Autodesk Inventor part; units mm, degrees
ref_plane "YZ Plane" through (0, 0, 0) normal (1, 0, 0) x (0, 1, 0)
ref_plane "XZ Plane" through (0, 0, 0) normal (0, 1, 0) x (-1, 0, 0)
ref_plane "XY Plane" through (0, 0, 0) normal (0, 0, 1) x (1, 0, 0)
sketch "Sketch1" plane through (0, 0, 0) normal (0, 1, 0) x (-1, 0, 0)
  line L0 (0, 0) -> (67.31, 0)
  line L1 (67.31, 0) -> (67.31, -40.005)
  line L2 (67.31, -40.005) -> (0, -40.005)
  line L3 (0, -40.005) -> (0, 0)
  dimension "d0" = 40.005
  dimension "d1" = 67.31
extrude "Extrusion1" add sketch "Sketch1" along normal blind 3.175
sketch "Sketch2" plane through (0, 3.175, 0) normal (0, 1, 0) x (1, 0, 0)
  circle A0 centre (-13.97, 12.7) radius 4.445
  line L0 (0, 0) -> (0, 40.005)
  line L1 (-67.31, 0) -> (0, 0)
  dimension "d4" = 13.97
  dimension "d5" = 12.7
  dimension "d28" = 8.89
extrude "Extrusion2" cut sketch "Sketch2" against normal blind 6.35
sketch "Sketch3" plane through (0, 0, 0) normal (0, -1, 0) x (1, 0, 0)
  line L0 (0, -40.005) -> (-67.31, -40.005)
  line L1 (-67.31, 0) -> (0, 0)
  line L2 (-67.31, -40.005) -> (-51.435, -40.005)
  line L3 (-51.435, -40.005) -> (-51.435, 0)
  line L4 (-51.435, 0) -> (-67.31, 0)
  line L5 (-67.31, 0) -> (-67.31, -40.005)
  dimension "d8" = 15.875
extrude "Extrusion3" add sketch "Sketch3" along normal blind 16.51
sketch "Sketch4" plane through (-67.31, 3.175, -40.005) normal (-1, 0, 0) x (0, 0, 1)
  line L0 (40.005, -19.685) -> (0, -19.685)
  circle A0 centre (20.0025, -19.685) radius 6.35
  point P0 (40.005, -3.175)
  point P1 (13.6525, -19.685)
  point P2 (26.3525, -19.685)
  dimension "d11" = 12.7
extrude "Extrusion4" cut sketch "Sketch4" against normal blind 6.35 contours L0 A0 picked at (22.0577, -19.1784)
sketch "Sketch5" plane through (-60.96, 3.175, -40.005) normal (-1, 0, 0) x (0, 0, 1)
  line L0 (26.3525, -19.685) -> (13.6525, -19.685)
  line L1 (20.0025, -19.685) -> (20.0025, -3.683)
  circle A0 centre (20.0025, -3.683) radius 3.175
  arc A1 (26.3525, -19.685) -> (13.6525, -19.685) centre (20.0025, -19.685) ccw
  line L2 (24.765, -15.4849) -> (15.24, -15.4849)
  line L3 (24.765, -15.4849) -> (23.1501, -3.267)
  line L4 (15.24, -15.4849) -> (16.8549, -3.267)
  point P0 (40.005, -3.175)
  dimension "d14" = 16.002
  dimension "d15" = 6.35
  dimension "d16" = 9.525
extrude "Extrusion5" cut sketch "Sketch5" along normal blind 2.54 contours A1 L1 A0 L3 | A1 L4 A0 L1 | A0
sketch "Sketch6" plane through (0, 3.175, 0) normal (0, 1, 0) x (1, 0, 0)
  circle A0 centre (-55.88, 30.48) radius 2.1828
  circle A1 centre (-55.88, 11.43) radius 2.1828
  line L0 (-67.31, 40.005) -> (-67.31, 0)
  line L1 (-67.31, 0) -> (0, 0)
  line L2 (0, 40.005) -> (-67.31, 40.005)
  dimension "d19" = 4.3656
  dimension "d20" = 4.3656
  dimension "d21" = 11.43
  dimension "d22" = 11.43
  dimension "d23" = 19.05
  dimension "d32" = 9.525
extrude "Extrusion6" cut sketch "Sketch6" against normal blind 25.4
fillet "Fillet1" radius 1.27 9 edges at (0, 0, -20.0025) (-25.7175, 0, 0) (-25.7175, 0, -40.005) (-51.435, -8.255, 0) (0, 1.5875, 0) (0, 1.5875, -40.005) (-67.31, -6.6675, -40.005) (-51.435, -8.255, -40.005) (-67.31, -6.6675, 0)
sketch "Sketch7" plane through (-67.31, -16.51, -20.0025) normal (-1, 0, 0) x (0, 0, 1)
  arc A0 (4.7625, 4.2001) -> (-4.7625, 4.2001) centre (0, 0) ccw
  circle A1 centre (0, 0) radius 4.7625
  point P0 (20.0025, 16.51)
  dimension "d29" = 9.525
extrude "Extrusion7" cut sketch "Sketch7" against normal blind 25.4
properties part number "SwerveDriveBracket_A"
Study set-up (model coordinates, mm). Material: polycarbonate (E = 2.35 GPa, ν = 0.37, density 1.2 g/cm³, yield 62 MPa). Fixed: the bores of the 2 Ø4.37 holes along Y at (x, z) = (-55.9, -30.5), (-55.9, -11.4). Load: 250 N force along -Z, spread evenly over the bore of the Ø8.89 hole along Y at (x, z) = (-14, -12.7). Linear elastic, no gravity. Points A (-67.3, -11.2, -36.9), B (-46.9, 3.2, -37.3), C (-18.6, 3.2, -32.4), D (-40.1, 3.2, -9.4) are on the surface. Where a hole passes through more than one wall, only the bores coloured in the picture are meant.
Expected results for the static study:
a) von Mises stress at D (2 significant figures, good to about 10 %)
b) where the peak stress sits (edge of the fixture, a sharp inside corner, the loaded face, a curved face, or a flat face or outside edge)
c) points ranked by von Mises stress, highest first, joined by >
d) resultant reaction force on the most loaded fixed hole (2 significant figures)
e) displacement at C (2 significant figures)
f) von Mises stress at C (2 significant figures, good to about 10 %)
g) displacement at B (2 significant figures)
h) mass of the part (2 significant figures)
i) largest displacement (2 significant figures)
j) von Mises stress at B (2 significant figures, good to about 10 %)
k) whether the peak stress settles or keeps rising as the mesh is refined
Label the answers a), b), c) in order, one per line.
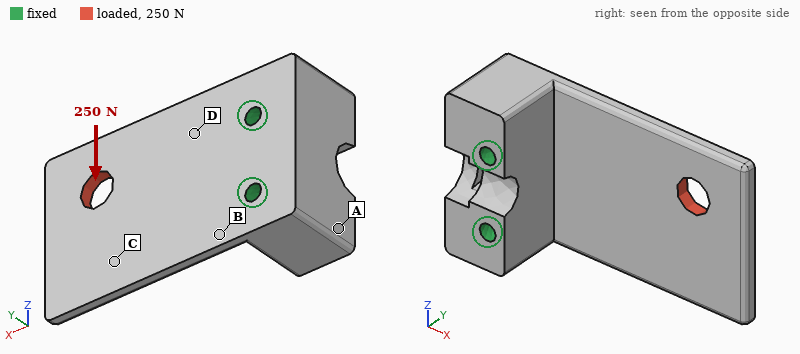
a) 5.2 MPa
b) edge of the fixture
c) B > D > C > A
d) 460 N
e) 0.26 mm
f) 2.6 MPa
g) 0.072 mm
h) 21 g
i) 0.42 mm
j) 7.2 MPa
k) keeps rising
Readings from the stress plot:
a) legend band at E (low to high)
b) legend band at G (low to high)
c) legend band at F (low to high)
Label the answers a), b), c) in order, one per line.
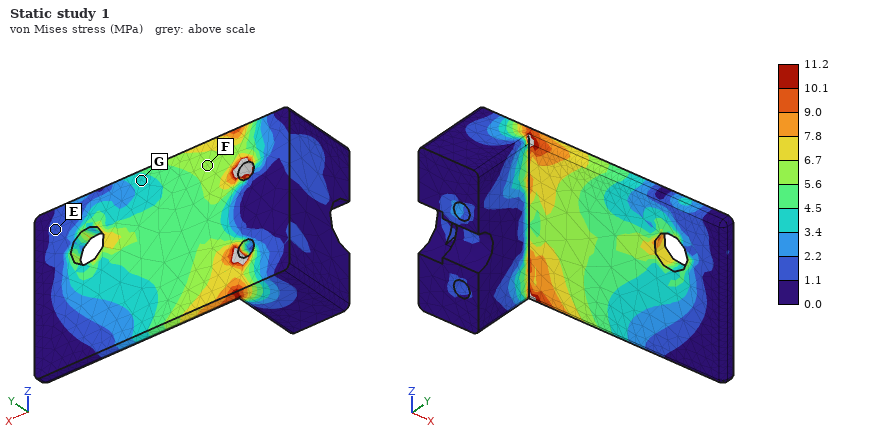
a) 1.1 to 2.2 MPa
b) 3.4 to 4.5 MPa
c) 5.6 to 6.7 MPa
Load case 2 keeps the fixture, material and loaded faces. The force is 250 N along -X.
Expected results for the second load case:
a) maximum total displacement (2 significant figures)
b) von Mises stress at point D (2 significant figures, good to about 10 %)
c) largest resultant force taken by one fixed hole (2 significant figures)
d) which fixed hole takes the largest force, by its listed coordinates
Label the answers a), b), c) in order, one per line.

a) 0.11 mm
b) 3.3 MPa
c) 220 N
d) (-55.9, -11.4)
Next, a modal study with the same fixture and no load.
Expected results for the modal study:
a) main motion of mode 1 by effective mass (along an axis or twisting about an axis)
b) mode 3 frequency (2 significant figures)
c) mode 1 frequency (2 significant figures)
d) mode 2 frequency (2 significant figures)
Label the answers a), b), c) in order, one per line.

a) along Y
b) 1600 Hz
c) 270 Hz
d) 760 Hz
